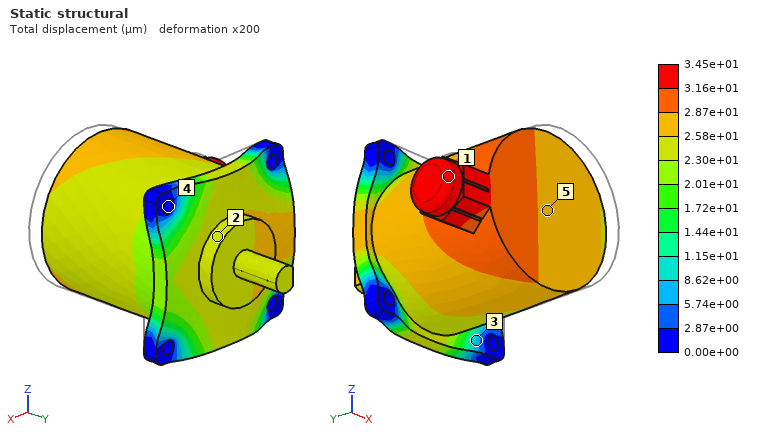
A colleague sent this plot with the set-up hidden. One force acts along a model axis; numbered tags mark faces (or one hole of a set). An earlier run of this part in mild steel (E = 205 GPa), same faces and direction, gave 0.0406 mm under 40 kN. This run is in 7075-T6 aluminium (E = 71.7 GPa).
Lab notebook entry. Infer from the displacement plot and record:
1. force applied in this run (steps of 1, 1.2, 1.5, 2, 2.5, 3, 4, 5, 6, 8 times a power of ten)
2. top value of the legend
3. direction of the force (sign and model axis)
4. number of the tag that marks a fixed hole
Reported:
12 kN
3.45e+01 µm
+Y
4
